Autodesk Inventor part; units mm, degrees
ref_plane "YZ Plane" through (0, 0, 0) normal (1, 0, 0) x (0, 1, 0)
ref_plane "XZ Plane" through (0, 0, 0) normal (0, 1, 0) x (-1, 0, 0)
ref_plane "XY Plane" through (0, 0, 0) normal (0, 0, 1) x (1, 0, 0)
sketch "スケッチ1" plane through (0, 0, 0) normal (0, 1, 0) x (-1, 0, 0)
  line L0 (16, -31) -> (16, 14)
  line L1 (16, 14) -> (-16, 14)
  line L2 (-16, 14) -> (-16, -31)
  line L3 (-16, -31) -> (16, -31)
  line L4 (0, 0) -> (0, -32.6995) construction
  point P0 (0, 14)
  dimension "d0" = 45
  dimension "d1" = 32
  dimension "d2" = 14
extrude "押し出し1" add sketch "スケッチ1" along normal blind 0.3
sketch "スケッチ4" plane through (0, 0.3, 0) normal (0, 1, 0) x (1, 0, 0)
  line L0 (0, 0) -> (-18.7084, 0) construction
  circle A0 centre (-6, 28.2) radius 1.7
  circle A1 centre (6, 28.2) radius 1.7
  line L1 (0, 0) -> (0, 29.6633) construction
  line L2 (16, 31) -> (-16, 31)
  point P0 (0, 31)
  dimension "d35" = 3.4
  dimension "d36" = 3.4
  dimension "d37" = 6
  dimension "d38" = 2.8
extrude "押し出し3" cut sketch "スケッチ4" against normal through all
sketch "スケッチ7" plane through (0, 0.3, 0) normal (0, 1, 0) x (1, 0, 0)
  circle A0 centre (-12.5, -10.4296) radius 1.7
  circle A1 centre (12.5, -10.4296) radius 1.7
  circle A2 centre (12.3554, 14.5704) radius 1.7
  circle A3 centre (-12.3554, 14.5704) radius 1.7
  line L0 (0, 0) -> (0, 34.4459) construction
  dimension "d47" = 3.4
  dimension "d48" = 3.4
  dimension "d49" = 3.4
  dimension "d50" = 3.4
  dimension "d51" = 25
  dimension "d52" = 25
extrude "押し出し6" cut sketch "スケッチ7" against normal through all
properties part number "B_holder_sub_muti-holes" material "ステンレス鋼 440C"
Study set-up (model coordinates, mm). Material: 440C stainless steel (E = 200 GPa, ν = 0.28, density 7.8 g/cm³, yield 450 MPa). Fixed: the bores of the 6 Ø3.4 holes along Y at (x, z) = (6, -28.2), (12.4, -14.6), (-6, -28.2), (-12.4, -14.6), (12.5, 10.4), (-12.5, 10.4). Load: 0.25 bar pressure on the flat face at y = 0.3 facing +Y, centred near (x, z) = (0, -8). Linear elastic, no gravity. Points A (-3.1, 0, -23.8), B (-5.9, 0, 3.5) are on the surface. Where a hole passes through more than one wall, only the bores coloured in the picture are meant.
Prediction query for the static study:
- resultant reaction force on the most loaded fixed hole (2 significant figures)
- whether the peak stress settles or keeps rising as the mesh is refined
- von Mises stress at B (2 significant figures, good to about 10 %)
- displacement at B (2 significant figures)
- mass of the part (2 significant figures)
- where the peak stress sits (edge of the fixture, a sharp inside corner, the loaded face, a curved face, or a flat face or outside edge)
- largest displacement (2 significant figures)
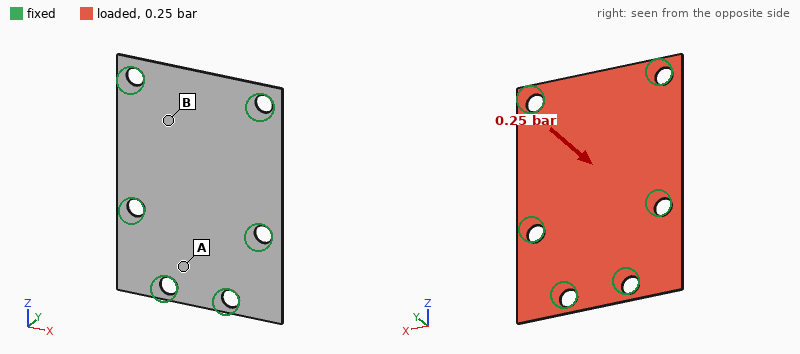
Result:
7.5 N
keeps rising
24 MPa
63 µm
3.2 g
edge of the fixture
95 µm
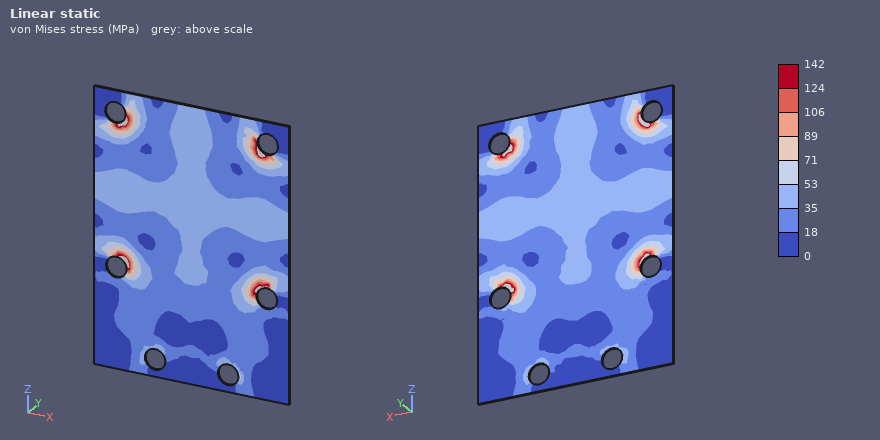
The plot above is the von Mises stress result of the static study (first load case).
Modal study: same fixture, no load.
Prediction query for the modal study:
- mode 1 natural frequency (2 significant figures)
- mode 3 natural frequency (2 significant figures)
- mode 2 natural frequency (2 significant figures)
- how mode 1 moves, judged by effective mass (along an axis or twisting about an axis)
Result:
2100 Hz
3500 Hz
3400 Hz
along Y
